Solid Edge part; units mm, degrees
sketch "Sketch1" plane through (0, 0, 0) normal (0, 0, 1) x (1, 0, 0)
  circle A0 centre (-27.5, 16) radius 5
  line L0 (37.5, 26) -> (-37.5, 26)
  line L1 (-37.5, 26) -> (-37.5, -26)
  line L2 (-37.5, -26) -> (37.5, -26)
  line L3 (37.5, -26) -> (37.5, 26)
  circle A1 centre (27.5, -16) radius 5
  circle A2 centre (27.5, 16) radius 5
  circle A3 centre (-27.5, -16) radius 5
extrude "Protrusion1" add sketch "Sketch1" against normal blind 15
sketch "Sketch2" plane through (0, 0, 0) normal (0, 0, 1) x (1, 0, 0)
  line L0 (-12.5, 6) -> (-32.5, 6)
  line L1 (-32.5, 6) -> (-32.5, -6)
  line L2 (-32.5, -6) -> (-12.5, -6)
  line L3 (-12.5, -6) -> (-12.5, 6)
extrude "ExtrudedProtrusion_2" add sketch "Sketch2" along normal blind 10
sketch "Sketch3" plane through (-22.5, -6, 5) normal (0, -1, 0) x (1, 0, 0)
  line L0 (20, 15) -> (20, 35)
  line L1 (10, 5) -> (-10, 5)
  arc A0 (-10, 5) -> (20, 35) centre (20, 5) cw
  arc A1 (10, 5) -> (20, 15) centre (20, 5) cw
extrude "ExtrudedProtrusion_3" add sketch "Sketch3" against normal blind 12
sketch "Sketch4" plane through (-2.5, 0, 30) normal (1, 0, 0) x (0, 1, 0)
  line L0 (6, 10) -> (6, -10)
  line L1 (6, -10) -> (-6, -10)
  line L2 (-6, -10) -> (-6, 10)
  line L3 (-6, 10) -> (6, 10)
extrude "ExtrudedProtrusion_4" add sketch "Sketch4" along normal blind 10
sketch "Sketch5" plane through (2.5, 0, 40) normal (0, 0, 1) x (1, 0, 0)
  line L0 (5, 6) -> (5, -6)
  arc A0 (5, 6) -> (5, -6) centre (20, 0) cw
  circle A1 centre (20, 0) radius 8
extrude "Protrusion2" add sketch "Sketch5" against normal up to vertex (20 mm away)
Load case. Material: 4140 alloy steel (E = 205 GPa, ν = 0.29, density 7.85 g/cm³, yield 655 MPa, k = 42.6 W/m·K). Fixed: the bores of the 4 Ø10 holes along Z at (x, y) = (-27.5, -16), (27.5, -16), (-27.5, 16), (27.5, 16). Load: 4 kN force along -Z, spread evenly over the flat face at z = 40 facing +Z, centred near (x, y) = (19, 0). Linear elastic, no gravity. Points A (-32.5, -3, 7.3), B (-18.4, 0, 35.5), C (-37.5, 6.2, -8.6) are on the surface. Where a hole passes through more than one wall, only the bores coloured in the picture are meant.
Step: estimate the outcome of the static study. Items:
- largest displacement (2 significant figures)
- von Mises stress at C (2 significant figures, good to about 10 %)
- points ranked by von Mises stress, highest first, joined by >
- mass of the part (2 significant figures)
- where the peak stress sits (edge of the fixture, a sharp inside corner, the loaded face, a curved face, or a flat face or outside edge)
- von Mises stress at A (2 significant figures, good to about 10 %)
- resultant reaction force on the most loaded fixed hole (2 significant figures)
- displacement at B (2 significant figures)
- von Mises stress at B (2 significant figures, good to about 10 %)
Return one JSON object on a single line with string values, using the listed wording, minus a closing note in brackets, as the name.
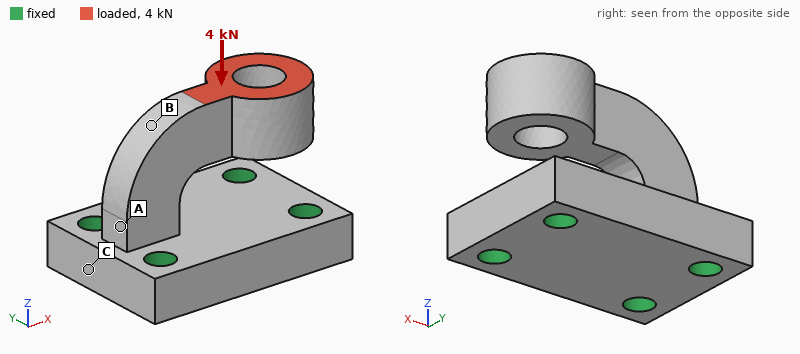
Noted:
{"largest displacement": "0.31 mm", "von Mises stress at C": "39 MPa", "points ranked by von Mises stress, highest first, joined by >": "A > B > C", "mass of the part": "610 g", "where the peak stress sits": "a curved face", "von Mises stress at A": "190 MPa", "resultant reaction force on the most loaded fixed hole": "1.1 kN", "displacement at B": "0.091 mm", "von Mises stress at B": "110 MPa"}
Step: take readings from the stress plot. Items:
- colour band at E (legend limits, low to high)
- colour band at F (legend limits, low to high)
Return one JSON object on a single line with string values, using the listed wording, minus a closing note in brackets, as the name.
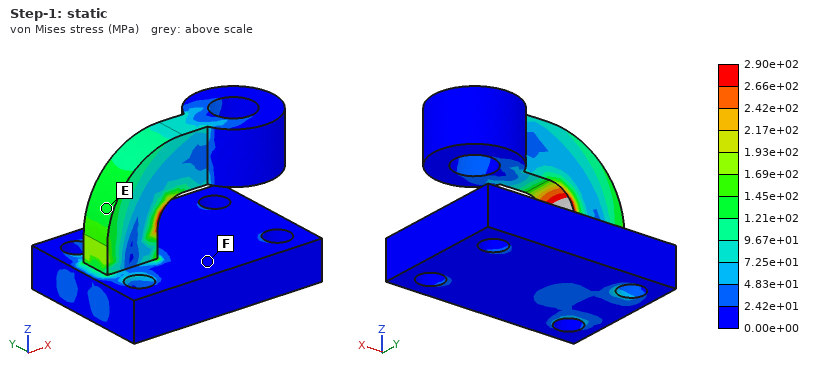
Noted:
{"colour band at E": "1.21e+02 to 1.45e+02 MPa", "colour band at F": "0.00e+00 to 2.42e+01 MPa"}
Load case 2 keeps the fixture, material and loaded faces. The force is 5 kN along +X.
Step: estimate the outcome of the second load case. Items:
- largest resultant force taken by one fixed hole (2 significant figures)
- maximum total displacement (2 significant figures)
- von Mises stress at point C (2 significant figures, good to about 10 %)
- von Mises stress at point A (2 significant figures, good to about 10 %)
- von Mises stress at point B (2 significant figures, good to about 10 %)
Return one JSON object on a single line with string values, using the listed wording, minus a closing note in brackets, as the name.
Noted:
{"largest resultant force taken by one fixed hole": "2.4 kN", "maximum total displacement": "0.27 mm", "von Mises stress at point C": "64 MPa", "von Mises stress at point A": "200 MPa", "von Mises stress at point B": "76 MPa"}
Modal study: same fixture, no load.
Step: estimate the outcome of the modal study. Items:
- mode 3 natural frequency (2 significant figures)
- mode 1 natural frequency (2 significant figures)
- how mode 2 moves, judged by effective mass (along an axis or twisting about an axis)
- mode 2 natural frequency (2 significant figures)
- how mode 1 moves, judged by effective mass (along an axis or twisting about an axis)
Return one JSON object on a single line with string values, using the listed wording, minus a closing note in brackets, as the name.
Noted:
{"mode 3 natural frequency": "3900 Hz", "mode 1 natural frequency": "1200 Hz", "how mode 2 moves, judged by effective mass": "along Z", "mode 2 natural frequency": "1900 Hz", "how mode 1 moves, judged by effective mass": "along Y"}
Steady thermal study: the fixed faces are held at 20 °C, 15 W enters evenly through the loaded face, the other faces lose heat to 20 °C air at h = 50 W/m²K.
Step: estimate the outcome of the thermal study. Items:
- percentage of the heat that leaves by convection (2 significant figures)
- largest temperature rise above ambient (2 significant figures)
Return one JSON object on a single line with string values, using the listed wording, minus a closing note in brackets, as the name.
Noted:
{"percentage of the heat that leaves by convection": "64 %", "largest temperature rise above ambient": "45 K"}
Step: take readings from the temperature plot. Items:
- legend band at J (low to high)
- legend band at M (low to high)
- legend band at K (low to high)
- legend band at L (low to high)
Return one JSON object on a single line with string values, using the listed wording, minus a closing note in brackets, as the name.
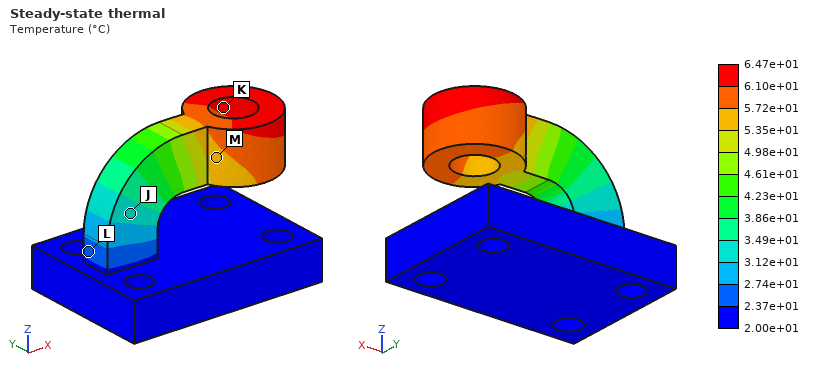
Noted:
{"legend band at J": "3.12e+01 to 3.49e+01 °C", "legend band at M": "5.35e+01 to 5.72e+01 °C", "legend band at K": "6.10e+01 to 6.47e+01 °C", "legend band at L": "2.37e+01 to 2.74e+01 °C"}
